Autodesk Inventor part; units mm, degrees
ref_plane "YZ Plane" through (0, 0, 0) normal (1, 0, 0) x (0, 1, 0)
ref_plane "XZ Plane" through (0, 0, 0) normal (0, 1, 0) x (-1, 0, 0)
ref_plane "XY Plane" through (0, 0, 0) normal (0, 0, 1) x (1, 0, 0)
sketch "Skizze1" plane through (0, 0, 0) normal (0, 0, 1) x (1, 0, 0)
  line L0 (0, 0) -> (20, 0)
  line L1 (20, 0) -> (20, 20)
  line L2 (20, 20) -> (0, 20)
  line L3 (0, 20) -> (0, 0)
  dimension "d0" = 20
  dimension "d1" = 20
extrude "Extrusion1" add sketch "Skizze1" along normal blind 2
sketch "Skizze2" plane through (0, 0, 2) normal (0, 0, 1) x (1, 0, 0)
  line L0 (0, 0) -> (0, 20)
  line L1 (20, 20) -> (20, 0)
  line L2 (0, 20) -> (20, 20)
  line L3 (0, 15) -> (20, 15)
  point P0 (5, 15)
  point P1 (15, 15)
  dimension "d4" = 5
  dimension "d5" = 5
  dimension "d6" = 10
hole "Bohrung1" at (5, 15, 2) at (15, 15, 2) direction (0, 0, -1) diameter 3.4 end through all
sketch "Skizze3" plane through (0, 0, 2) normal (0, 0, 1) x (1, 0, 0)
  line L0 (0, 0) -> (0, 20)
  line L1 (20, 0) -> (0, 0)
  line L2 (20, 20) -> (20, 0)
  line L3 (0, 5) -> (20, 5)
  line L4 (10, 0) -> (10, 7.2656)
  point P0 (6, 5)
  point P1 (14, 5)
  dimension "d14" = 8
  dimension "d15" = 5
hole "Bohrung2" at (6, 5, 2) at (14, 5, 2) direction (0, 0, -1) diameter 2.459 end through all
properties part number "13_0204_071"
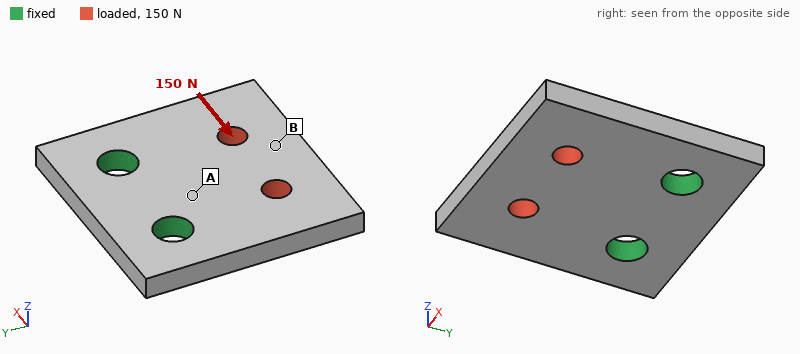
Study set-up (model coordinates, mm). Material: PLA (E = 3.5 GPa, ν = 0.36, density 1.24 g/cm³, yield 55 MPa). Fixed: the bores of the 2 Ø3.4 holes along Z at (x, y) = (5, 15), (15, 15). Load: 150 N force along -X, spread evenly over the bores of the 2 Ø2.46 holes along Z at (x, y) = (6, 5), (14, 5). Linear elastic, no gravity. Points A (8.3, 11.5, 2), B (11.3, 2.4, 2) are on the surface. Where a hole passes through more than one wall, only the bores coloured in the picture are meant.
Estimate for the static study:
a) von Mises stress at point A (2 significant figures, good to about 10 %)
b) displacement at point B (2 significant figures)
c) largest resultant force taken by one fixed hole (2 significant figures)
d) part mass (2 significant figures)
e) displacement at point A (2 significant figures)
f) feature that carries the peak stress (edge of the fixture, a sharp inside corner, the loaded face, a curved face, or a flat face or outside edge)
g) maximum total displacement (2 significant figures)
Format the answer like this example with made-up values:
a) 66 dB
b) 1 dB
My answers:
a) 10.0 MPa
b) 57 µm
c) 130 N
d) 0.92 g
e) 11 µm
f) edge of the fixture
g) 68 µm
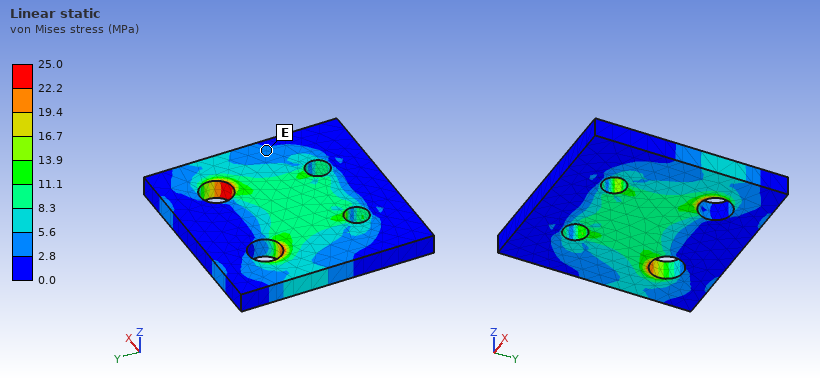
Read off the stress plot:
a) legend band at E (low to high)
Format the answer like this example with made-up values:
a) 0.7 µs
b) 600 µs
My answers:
a) 2.8 to 5.6 MPa
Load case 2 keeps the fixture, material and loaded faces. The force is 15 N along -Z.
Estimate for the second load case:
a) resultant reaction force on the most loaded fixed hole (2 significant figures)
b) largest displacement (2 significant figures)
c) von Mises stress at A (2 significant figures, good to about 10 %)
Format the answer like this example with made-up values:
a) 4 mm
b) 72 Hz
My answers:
a) 7.5 N
b) 0.15 mm
c) 6.1 MPa
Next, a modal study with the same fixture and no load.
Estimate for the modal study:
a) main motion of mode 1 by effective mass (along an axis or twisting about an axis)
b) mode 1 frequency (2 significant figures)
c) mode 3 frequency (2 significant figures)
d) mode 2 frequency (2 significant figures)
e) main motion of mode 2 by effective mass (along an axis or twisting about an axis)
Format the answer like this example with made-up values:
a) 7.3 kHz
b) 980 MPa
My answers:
a) along Z
b) 2800 Hz
c) 11 kHz
d) 4800 Hz
e) twisting about Y
